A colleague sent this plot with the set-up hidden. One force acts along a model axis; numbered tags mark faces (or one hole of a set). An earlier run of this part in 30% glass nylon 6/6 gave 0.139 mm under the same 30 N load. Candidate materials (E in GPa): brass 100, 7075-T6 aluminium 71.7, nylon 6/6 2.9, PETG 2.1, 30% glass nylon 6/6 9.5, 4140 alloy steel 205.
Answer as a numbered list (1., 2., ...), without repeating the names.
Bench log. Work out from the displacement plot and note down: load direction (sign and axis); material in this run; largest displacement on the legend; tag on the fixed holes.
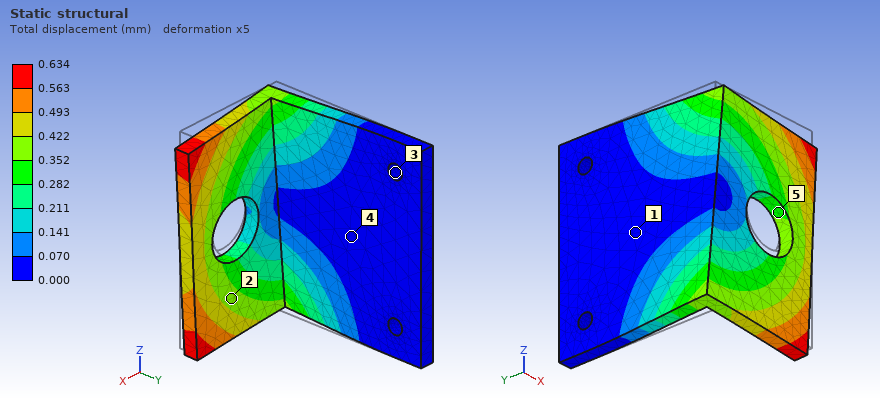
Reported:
1. -Z
2. PETG
3. 0.634 mm
4. 3
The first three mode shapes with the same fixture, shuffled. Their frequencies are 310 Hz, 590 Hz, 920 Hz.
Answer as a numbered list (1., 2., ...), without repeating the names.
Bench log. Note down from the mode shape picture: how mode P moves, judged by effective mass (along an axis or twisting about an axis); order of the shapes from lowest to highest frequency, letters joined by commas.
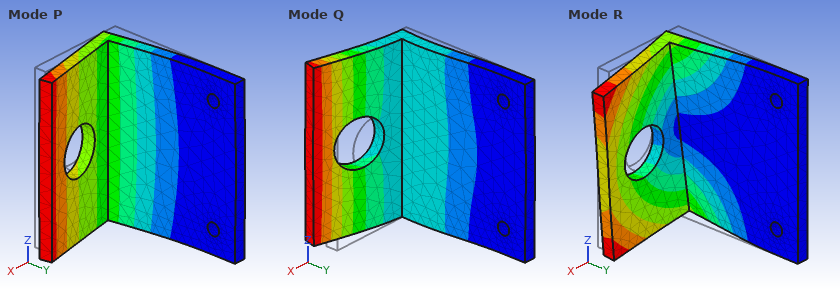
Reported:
1. along X
2. P, R, Q
